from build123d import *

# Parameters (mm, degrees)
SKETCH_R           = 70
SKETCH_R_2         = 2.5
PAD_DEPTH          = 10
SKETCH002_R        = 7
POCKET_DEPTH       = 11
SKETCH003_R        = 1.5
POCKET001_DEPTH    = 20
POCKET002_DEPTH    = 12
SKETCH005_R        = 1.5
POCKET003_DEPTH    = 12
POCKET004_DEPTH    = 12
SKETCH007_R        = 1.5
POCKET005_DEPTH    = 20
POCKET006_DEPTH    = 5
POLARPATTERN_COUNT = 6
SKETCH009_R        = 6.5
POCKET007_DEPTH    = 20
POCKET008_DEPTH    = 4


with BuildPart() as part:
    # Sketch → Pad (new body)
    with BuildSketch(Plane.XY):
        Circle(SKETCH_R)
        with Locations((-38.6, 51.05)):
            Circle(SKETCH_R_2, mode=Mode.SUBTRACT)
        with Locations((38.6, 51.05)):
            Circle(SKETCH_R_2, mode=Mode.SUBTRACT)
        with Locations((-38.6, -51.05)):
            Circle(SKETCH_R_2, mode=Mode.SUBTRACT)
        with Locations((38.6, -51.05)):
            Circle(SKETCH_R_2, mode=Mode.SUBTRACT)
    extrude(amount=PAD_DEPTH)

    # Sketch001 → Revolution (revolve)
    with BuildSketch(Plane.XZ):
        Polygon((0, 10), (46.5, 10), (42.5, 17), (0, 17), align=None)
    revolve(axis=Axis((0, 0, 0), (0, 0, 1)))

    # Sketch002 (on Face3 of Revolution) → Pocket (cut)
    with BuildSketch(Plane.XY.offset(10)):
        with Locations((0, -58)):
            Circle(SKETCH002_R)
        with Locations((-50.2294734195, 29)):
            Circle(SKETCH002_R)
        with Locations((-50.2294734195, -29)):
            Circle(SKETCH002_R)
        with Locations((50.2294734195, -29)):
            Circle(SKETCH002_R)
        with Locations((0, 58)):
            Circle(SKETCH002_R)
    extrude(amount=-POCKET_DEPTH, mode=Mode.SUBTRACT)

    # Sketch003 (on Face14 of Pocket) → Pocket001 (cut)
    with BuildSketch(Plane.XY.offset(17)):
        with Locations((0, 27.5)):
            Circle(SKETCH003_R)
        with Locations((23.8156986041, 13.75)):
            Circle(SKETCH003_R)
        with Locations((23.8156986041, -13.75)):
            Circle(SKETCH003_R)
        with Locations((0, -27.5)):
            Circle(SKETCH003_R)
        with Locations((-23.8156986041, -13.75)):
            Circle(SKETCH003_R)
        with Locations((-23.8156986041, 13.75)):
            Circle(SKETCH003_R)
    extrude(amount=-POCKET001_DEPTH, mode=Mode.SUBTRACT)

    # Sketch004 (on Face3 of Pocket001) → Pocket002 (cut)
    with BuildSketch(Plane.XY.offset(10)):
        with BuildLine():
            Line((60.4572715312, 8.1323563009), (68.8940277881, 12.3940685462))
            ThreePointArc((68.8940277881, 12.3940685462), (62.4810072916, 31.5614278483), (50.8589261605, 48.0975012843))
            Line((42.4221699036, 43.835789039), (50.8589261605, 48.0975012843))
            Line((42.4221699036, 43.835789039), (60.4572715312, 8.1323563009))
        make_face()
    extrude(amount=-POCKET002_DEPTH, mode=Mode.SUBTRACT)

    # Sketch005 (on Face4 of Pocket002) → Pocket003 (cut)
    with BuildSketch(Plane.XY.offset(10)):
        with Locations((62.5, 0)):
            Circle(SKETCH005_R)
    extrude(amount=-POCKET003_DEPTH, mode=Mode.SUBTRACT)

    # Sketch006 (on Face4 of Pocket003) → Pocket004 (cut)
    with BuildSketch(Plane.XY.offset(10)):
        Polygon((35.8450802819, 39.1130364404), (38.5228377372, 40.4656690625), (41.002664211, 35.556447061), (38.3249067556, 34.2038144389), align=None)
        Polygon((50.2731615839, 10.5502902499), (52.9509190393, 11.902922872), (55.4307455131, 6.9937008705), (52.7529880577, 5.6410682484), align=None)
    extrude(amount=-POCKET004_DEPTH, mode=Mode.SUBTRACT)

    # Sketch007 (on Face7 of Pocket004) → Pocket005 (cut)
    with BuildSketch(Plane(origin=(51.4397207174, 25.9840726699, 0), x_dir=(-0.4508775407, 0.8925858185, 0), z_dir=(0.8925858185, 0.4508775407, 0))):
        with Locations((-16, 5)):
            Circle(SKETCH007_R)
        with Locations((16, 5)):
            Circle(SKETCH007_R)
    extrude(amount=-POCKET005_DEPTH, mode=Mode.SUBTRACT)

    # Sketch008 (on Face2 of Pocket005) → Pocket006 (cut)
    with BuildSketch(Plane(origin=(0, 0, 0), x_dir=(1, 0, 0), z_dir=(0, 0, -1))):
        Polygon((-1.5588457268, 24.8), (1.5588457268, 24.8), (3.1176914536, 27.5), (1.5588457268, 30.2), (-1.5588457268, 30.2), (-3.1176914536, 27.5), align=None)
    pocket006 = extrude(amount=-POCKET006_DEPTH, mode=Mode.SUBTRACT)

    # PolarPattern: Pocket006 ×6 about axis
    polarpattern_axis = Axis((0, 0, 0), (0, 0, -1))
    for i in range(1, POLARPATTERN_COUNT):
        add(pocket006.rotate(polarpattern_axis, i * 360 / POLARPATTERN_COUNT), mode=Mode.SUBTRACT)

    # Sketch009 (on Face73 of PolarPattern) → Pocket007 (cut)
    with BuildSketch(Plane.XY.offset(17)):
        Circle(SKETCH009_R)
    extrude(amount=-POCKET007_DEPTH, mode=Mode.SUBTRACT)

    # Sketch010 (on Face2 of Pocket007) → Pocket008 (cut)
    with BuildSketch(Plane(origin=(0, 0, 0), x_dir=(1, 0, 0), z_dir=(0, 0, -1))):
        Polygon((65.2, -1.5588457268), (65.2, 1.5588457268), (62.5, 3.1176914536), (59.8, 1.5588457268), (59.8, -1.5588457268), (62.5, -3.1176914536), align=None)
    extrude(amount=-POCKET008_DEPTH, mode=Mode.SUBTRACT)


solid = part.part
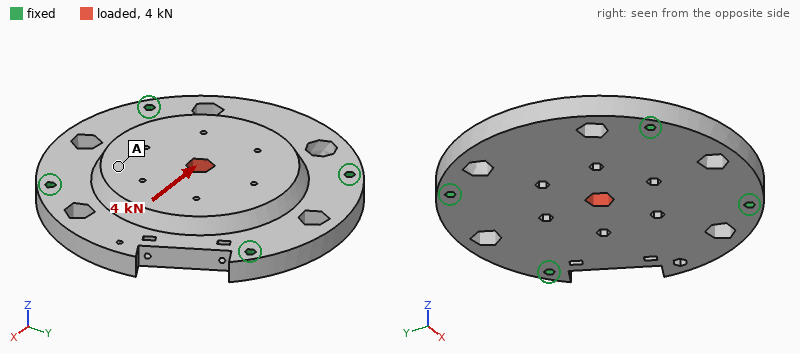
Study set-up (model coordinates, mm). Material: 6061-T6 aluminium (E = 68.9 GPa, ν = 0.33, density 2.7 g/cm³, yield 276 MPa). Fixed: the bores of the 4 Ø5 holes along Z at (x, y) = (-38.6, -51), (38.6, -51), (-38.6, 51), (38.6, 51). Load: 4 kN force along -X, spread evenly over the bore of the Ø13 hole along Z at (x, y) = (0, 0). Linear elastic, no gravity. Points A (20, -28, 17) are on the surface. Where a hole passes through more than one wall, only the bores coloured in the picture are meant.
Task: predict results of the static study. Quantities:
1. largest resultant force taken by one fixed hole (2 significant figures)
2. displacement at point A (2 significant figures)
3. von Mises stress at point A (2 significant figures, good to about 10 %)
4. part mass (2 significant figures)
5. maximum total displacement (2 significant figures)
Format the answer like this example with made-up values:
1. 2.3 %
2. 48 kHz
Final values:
1. 1.1 kN
2. 2.8 µm
3. 2.2 MPa
4. 490 g
5. 5.0 µm
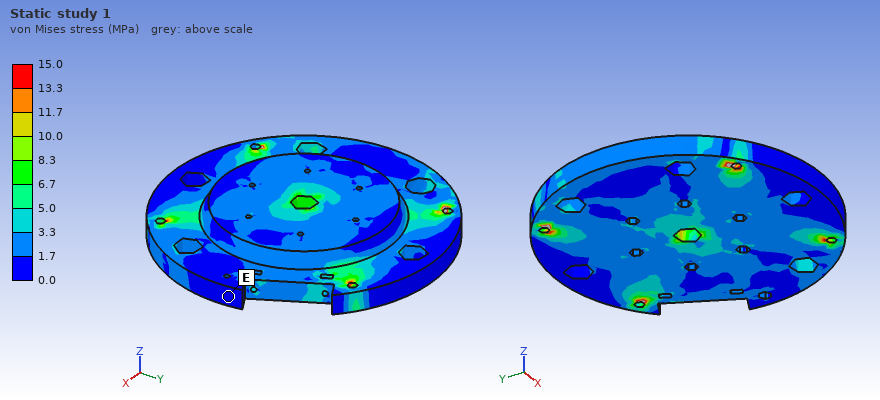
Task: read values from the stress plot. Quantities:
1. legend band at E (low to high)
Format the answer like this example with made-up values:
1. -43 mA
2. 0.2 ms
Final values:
1. 0.0 to 1.7 MPa
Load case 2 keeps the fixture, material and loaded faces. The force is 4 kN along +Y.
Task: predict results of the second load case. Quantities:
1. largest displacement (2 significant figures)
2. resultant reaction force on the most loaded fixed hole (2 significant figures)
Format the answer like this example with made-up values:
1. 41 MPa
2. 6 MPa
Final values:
1. 4.0 µm
2. 1.1 kN
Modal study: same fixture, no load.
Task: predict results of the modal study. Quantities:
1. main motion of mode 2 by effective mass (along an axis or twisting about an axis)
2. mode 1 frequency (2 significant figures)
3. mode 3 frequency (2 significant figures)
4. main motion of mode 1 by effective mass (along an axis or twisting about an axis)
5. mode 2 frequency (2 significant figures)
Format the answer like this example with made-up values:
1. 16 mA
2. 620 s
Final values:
1. twisting about Y
2. 3800 Hz
3. 6000 Hz
4. along Z
5. 4200 Hz
